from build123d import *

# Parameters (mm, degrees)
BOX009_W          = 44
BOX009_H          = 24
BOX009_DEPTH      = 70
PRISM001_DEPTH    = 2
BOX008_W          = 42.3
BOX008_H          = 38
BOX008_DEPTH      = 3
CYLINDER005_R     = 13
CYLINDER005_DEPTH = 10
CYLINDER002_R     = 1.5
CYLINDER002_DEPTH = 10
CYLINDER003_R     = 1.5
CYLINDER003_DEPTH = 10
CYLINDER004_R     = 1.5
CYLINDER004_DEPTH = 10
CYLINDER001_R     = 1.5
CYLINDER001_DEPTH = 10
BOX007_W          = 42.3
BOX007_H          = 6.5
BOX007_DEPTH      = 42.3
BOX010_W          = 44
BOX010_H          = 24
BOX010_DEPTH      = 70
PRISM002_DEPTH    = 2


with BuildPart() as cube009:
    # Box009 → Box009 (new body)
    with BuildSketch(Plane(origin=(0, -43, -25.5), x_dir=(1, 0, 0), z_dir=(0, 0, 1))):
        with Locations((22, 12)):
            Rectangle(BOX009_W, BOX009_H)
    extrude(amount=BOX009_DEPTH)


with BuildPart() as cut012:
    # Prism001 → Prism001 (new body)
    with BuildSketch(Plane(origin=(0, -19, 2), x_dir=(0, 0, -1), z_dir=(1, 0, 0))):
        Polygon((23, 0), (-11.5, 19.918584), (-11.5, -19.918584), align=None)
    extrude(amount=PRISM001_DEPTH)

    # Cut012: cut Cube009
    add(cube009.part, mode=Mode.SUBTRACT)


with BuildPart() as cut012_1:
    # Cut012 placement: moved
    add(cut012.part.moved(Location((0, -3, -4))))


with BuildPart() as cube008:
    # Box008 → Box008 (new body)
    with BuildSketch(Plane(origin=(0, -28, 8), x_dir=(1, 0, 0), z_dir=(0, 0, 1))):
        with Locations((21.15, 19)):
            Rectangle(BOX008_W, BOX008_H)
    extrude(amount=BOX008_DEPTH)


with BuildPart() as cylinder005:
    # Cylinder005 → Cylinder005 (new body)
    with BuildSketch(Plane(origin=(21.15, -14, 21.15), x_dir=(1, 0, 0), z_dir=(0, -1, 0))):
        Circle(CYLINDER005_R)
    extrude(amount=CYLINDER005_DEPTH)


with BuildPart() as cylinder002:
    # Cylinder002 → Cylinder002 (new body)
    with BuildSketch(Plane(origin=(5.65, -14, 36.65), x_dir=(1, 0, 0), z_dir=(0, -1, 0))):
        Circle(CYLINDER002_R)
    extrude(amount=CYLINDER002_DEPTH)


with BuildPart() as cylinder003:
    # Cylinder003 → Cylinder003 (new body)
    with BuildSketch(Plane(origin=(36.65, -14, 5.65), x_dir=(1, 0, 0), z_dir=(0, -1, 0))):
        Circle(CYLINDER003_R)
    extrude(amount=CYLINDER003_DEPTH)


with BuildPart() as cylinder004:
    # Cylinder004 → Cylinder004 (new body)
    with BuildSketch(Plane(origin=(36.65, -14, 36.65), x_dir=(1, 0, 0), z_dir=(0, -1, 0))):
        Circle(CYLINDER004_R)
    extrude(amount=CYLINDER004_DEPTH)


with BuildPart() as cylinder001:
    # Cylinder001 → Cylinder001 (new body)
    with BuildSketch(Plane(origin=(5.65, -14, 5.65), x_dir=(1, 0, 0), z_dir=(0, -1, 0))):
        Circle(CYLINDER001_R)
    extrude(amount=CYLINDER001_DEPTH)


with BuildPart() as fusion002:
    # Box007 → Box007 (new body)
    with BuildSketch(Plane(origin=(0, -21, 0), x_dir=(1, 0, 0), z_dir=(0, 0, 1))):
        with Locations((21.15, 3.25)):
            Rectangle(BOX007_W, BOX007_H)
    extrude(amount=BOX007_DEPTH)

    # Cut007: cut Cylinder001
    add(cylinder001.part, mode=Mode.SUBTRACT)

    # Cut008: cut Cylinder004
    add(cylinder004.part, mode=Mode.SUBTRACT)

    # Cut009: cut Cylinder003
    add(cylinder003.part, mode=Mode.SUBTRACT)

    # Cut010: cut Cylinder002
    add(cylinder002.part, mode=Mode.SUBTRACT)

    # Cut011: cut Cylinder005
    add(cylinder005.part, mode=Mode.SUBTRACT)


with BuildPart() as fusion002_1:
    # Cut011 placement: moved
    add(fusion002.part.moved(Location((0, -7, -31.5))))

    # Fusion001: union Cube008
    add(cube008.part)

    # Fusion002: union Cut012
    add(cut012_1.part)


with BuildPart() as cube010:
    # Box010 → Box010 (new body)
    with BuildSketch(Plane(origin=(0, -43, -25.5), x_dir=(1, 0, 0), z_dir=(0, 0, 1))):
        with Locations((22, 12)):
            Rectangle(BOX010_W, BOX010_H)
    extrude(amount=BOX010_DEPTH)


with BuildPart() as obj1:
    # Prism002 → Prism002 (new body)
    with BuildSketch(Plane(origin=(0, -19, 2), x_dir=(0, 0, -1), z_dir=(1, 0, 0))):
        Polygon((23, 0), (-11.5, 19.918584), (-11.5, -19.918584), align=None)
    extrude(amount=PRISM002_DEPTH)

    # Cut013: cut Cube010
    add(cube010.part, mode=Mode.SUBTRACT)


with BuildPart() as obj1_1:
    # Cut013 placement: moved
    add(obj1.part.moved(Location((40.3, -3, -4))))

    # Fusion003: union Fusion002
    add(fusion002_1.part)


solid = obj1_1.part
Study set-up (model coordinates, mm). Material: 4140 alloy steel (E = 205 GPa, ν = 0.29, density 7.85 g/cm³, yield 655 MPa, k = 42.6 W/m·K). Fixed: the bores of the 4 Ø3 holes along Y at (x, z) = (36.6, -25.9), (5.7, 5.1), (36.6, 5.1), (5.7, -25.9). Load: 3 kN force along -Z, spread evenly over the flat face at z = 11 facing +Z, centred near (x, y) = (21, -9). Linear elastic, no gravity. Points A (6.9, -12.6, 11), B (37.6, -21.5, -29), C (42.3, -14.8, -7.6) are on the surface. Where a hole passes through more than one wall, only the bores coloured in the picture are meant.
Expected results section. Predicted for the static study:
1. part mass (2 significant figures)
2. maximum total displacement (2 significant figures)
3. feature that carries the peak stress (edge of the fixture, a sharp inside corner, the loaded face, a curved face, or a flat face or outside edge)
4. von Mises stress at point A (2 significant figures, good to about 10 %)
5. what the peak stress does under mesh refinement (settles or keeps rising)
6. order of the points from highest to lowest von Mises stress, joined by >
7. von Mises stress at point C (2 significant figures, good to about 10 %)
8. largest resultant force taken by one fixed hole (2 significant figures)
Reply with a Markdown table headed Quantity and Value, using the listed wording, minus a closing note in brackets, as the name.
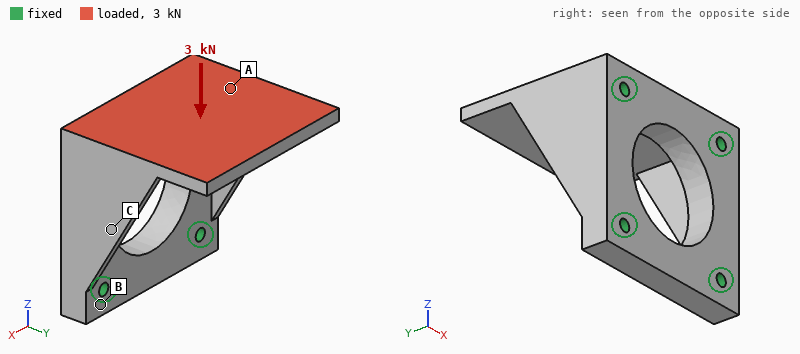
| Quantity | Value |
|---|---|
| part mass | 100 g |
| maximum total displacement | 0.19 mm |
| feature that carries the peak stress | a sharp inside corner |
| von Mises stress at point A | 140 MPa |
| what the peak stress does under mesh refinement | keeps rising |
| order of the points from highest to lowest von Mises stress, joined by > | A > C > B |
| von Mises stress at point C | 80 MPa |
| largest resultant force taken by one fixed hole | 1.3 kN |
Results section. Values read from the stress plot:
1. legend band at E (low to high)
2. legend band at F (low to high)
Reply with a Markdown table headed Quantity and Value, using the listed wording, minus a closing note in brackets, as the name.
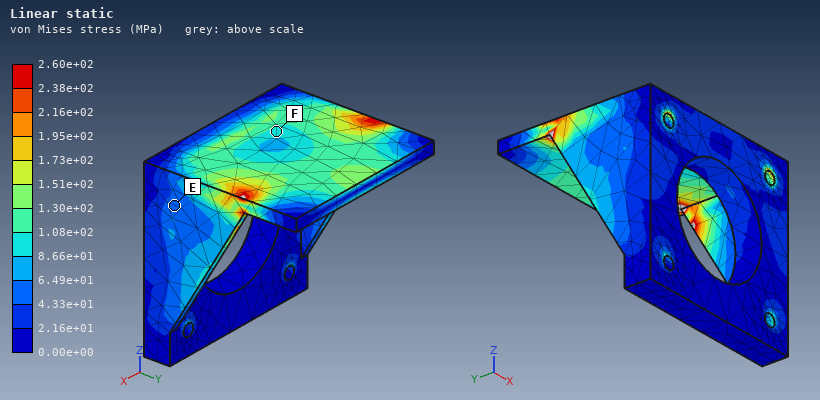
| Quantity | Value |
|---|---|
| legend band at E | 4.33e+01 to 6.49e+01 MPa |
| legend band at F | 8.66e+01 to 1.08e+02 MPa |
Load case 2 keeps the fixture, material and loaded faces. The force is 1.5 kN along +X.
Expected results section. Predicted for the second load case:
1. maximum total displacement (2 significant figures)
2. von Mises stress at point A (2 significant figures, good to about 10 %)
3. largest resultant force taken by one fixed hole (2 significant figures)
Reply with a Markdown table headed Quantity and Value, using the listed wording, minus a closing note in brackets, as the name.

| Quantity | Value |
|---|---|
| maximum total displacement | 5.6 µm |
| von Mises stress at point A | 12 MPa |
| largest resultant force taken by one fixed hole | 1.0 kN |
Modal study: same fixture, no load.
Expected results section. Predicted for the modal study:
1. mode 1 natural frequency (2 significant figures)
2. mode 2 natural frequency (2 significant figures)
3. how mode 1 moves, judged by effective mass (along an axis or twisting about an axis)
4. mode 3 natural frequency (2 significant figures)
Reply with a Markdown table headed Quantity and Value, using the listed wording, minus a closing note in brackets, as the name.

| Quantity | Value |
|---|---|
| mode 1 natural frequency | 4300 Hz |
| mode 2 natural frequency | 9200 Hz |
| how mode 1 moves, judged by effective mass | along Z |
| mode 3 natural frequency | 14 kHz |
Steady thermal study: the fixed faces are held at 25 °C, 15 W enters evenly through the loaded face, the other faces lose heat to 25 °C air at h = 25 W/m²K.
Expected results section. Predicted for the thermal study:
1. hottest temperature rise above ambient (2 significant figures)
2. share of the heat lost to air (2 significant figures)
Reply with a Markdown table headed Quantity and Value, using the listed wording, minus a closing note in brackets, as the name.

| Quantity | Value |
|---|---|
| hottest temperature rise above ambient | 37 K |
| share of the heat lost to air | 11 % |
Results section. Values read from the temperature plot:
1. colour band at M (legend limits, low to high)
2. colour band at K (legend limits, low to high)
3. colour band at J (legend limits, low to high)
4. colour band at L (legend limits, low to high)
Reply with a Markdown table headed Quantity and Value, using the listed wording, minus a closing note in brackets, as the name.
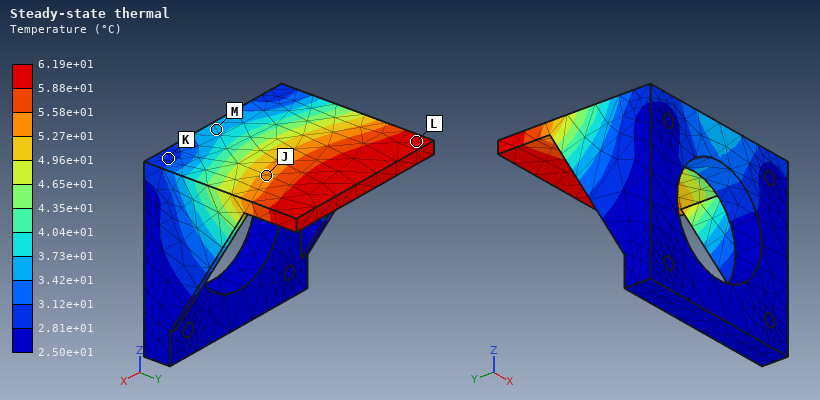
| Quantity | Value |
|---|---|
| colour band at M | 3.42e+01 to 3.73e+01 °C |
| colour band at K | 2.81e+01 to 3.12e+01 °C |
| colour band at J | 5.27e+01 to 5.58e+01 °C |
| colour band at L | 5.88e+01 to 6.19e+01 °C |
